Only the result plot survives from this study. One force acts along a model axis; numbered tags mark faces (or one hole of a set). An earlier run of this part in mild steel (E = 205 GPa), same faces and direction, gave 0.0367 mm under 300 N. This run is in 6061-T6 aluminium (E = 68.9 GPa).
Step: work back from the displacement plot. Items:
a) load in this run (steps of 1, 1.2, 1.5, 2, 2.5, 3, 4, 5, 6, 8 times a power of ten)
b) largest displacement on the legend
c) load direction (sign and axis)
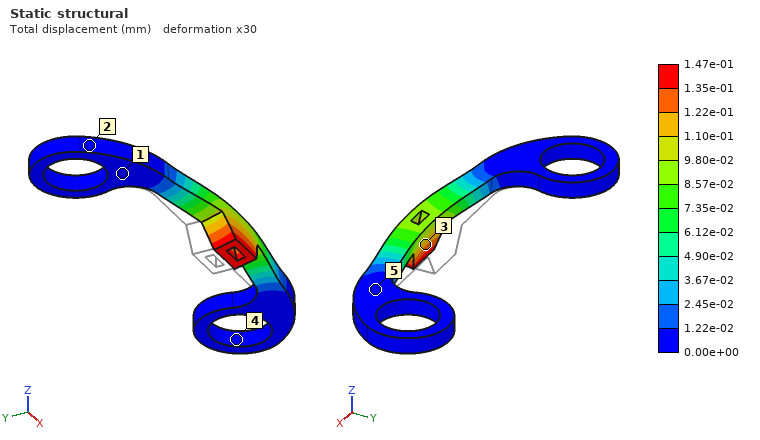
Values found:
400 N
1.47e-01 mm
-Y
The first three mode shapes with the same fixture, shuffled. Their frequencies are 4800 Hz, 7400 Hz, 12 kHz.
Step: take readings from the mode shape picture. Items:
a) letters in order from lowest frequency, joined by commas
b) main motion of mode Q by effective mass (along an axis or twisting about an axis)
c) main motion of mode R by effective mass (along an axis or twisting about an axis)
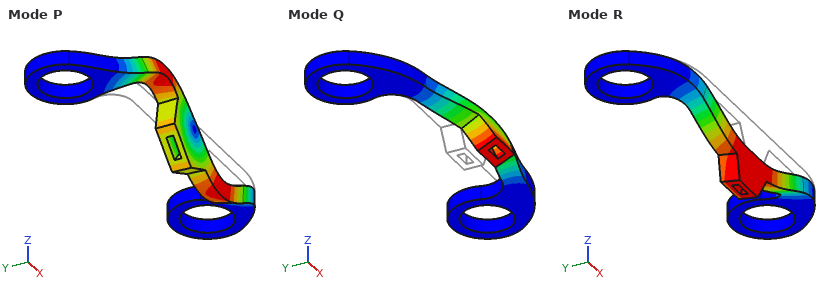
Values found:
R, Q, P
along Y
along Z
